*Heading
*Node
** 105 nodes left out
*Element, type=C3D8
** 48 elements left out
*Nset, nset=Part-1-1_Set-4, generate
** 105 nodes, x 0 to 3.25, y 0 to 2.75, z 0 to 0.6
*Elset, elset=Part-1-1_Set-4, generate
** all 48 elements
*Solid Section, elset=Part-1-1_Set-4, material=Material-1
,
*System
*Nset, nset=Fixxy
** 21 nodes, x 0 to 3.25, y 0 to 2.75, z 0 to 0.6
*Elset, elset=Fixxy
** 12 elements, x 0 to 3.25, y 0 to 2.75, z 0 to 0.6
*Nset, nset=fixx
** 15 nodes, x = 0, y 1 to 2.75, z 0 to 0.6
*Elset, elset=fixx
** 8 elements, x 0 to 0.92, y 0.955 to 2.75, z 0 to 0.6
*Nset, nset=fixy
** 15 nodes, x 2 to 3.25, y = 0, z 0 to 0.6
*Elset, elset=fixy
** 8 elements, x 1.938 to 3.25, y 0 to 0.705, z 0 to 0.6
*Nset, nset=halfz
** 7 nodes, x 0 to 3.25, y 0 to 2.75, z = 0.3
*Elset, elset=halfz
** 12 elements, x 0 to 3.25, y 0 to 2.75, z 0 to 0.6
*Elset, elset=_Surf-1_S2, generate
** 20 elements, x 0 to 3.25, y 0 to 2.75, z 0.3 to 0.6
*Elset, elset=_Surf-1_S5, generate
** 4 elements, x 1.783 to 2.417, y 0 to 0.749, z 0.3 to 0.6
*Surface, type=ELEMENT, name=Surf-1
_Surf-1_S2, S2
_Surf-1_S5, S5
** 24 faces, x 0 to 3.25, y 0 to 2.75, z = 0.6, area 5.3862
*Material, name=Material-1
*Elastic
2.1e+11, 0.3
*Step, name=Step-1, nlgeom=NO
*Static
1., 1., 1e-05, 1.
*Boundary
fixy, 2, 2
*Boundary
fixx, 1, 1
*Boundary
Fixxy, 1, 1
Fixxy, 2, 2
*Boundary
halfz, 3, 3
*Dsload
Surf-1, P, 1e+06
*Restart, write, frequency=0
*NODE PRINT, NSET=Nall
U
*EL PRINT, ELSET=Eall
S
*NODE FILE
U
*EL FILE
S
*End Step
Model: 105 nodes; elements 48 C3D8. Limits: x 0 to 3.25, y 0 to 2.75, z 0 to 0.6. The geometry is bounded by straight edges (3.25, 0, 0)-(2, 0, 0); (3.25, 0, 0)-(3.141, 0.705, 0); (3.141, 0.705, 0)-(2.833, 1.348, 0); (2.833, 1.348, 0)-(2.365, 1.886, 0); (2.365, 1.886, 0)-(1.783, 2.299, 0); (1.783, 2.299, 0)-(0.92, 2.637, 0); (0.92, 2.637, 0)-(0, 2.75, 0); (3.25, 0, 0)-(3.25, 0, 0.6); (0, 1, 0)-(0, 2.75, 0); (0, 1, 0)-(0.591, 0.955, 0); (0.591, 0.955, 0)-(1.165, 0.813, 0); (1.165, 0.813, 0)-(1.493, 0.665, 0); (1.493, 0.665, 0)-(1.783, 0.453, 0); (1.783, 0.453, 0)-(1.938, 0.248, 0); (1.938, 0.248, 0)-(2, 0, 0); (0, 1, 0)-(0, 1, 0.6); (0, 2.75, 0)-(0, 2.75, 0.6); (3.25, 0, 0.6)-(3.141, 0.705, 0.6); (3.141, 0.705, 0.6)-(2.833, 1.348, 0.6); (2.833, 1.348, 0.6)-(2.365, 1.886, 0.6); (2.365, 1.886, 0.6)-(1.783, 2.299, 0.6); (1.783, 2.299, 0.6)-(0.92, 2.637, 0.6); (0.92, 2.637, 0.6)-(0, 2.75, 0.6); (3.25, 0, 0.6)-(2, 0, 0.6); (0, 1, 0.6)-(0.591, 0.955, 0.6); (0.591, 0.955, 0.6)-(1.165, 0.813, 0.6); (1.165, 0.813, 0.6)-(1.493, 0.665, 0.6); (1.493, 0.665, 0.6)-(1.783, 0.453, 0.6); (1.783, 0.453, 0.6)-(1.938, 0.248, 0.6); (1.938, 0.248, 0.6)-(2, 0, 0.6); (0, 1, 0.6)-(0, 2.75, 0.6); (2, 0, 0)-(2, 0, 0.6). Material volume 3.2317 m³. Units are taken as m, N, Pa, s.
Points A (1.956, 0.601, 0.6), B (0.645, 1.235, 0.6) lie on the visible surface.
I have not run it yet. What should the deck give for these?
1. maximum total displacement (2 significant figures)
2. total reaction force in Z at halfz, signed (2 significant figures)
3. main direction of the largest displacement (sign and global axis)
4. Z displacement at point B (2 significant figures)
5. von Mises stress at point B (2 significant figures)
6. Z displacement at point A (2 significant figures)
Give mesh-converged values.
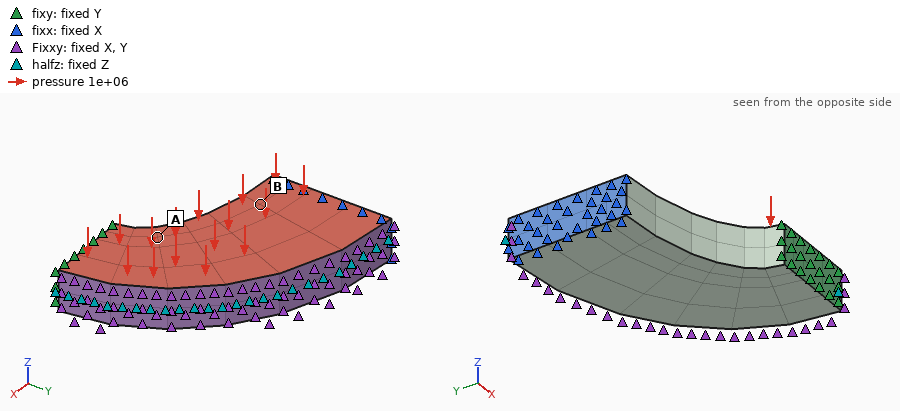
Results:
2.0e-04 m
5.4e+06 N
-Z
-1.5e-04 m
4.1e+06 Pa
-9.2e-05 m
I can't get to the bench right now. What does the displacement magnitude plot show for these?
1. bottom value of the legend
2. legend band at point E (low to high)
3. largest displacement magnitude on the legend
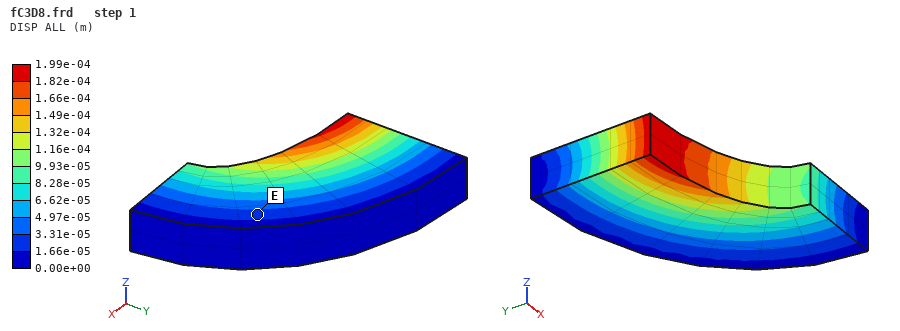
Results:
0.00e+00 m
1.66e-05 to 3.31e-05 m
1.99e-04 m
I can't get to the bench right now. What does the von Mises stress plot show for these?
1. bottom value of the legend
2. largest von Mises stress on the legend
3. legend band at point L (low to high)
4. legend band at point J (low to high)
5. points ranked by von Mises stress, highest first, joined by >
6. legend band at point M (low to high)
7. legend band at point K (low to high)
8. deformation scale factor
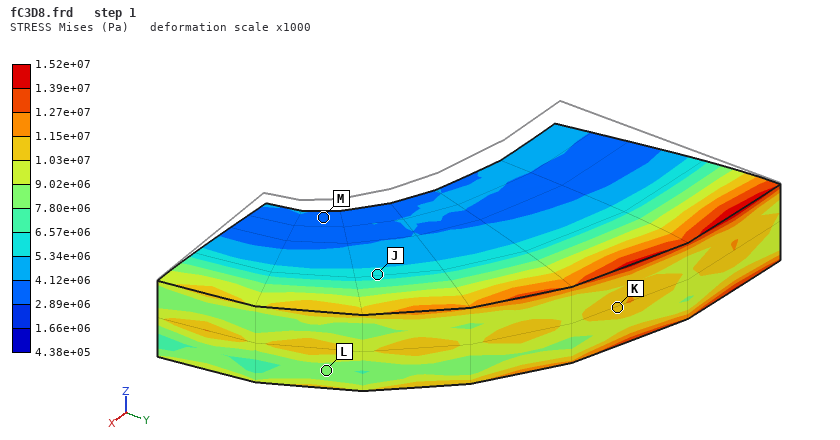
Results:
4.38e+05 Pa
1.52e+07 Pa
7.80e+06 to 9.02e+06 Pa
5.34e+06 to 6.57e+06 Pa
K > L > J > M
2.89e+06 to 4.12e+06 Pa
1.03e+07 to 1.15e+07 Pa
1000
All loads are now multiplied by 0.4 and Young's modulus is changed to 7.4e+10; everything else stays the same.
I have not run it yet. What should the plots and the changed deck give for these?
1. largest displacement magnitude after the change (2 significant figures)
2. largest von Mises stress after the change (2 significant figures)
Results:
2.3e-04 m
6.1e+06 Pa
